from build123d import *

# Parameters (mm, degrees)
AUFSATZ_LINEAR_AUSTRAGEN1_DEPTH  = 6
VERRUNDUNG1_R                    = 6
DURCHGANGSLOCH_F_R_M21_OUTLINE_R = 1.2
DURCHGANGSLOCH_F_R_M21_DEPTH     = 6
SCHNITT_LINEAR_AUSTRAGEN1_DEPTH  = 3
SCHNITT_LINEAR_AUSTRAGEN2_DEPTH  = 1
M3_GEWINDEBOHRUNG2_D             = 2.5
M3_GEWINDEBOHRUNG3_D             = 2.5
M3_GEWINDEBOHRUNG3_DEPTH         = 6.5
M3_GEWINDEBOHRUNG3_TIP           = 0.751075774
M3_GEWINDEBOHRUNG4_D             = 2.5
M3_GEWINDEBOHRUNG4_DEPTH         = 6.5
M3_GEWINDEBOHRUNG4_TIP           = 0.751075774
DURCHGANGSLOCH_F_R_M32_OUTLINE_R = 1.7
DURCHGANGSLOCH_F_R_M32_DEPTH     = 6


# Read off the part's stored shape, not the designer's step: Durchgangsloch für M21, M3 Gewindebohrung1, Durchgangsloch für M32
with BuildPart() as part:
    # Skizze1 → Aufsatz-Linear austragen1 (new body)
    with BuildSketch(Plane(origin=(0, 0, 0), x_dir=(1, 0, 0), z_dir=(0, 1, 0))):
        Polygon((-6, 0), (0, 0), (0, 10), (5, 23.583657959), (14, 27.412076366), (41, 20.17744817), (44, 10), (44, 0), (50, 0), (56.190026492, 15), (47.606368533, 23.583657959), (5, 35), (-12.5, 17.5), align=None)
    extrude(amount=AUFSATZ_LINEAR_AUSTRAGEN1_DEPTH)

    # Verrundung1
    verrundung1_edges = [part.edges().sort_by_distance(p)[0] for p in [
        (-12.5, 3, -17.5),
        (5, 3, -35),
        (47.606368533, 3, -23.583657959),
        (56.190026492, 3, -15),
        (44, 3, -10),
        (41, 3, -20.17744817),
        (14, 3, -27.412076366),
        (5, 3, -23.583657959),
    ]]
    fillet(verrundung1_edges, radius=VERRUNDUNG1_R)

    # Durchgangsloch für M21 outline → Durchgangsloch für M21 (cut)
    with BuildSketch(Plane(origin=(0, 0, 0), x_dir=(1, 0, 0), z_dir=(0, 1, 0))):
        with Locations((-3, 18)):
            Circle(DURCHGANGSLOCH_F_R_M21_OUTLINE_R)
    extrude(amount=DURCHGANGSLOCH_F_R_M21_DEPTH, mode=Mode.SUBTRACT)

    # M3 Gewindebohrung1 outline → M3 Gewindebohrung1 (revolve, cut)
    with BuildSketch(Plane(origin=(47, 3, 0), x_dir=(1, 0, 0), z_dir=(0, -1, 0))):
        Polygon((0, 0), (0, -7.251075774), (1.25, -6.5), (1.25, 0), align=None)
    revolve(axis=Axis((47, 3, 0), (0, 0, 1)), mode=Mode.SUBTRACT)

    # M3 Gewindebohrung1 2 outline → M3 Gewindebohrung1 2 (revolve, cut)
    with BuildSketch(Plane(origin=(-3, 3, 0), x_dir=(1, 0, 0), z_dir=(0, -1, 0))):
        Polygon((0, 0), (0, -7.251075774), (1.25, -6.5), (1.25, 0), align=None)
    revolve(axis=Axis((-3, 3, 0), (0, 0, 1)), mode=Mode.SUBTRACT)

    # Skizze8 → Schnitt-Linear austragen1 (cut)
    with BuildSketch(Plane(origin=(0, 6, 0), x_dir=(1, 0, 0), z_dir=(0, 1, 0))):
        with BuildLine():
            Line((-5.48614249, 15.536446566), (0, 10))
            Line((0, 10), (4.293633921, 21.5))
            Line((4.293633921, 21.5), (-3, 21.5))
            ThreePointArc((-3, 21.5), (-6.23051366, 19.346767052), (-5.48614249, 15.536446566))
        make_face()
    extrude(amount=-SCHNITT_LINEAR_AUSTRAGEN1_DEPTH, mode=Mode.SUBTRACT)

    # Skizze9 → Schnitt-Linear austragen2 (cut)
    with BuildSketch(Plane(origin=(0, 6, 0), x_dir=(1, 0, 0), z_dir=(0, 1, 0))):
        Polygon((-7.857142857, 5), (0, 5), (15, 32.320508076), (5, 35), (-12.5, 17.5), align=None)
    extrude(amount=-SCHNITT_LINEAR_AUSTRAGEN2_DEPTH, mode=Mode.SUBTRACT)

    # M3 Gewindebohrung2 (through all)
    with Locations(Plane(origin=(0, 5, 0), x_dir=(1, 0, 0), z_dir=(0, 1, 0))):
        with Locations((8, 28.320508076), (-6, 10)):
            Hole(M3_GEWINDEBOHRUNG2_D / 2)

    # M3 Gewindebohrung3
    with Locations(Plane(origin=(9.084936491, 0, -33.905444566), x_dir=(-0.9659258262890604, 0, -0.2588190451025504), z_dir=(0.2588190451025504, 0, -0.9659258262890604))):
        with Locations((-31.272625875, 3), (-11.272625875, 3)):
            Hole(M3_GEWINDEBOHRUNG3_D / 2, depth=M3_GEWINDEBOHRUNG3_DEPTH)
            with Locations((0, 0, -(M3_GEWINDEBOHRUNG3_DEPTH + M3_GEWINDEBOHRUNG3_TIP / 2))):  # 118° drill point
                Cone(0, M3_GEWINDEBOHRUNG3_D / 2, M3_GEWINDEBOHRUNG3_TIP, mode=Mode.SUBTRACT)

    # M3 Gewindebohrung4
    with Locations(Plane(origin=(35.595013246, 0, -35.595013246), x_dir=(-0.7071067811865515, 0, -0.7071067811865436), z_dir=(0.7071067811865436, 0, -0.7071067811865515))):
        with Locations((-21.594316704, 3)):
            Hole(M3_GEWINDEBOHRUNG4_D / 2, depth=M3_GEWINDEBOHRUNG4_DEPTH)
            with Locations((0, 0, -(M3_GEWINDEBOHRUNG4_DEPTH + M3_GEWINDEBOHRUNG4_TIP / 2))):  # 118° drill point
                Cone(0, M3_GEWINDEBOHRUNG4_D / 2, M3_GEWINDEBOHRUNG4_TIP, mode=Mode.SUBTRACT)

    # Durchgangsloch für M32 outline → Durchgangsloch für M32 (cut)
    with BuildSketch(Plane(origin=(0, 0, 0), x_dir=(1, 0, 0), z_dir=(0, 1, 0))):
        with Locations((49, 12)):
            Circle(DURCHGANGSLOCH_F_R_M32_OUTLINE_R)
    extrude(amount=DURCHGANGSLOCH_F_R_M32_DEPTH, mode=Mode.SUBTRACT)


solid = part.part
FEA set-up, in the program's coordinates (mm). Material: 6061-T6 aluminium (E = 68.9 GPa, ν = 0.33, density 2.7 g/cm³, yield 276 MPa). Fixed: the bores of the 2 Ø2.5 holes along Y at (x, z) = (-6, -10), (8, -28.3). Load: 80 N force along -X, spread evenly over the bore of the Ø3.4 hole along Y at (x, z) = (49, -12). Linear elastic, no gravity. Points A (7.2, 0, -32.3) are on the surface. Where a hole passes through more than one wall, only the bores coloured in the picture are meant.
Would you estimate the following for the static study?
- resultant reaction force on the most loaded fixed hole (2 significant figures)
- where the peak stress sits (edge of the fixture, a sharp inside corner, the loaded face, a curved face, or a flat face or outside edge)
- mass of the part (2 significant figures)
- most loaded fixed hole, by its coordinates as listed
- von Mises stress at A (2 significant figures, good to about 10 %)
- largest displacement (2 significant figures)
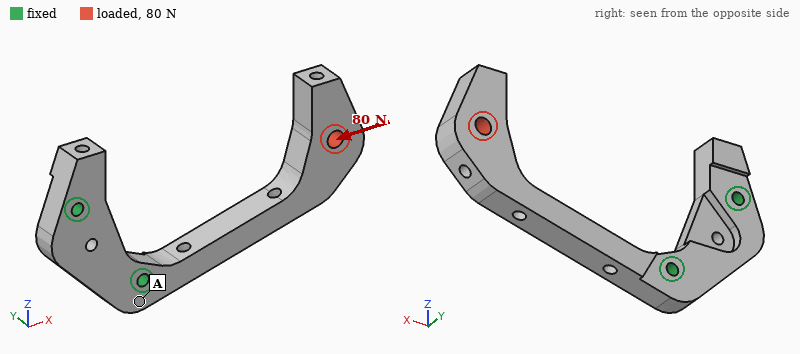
100 N
a curved face
10 g
(8, -28.3)
11 MPa
0.38 mm
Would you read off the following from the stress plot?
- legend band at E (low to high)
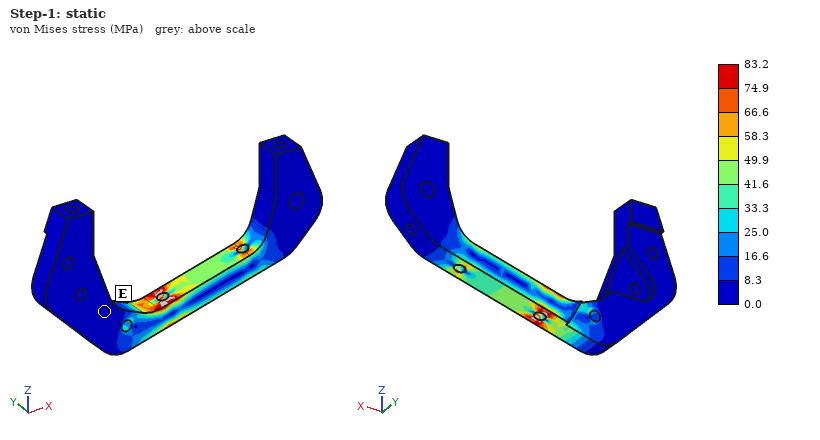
0.0 to 8.3 MPa
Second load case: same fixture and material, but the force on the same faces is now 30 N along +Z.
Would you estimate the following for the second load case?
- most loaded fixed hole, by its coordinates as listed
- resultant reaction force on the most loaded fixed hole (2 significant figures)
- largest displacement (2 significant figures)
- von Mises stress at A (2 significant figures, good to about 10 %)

(8, -28.3)
83 N
0.23 mm
10 MPa
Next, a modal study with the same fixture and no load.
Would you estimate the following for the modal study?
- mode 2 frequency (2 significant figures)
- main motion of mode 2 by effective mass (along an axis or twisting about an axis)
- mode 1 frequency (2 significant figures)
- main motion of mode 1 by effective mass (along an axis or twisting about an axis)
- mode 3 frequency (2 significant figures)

1100 Hz
along Y
1000 Hz
along Z
4000 Hz
